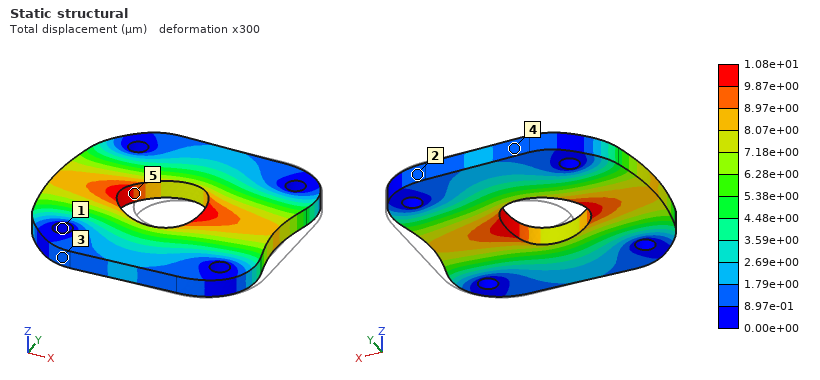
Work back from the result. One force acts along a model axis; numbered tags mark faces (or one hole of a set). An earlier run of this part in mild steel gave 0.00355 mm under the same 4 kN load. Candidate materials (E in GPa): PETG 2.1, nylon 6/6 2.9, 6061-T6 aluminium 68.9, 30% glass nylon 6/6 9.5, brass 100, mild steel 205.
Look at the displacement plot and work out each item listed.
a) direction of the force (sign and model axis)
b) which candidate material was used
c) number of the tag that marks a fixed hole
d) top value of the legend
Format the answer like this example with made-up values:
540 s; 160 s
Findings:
-X; 6061-T6 aluminium; 1; 1.08e+01 µm
